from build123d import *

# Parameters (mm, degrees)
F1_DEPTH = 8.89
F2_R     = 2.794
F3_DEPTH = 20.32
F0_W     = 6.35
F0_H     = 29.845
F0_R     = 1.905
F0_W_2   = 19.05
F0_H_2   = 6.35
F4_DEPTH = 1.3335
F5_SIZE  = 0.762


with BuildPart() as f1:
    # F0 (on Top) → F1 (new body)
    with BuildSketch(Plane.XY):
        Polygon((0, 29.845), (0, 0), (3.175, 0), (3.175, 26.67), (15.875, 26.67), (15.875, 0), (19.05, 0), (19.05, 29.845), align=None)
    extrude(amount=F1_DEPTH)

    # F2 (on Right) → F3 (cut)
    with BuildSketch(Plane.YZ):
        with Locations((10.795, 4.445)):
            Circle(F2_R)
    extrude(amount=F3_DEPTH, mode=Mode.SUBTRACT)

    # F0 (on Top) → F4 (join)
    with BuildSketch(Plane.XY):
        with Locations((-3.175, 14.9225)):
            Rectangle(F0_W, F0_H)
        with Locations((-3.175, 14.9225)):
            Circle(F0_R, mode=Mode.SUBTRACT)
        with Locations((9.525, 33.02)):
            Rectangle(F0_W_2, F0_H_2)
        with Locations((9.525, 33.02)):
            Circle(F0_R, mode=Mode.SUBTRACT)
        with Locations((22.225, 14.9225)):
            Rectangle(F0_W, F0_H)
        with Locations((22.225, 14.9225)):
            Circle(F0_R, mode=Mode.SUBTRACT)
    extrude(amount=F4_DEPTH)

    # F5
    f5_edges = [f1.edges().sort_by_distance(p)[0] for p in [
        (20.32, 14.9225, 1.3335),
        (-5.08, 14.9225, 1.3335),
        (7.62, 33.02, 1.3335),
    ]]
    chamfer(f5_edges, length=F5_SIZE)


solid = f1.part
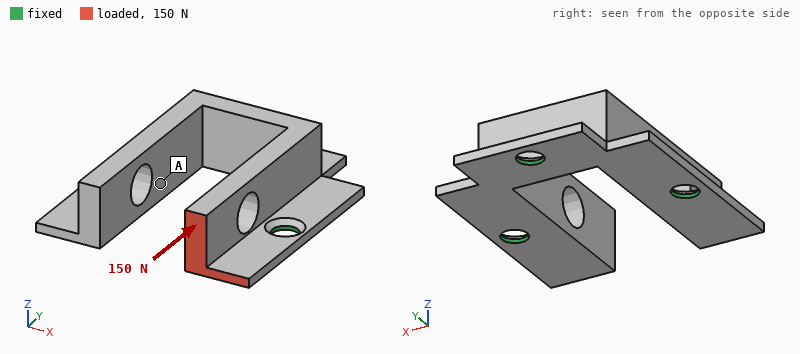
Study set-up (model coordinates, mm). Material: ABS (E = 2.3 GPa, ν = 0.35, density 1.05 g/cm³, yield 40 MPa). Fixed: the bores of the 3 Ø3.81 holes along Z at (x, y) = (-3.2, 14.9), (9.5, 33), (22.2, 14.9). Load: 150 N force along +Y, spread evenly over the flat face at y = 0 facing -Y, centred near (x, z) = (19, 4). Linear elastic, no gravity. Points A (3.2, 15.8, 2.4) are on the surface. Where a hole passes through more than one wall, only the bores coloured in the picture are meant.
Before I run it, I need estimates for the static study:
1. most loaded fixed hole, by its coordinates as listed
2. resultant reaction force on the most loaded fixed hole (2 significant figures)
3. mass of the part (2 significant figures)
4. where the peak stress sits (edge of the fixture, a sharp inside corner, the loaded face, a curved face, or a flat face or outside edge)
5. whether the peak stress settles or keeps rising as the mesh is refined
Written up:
(22.2, 14.9)
120 N
2.6 g
edge of the fixture
keeps rising
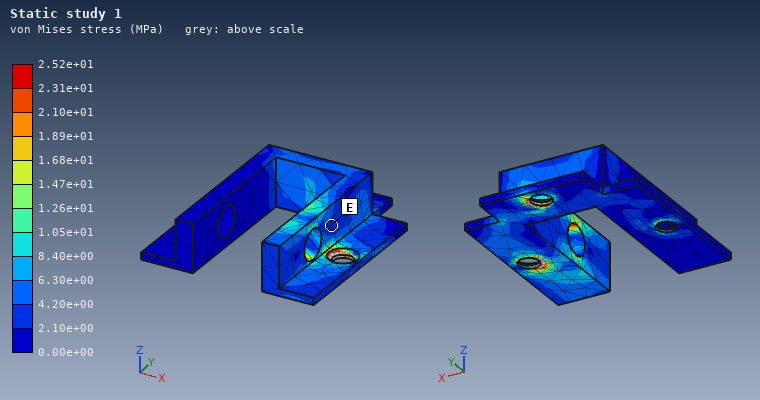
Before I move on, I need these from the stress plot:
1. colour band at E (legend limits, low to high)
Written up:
2.10e+00 to 4.20e+00 MPa
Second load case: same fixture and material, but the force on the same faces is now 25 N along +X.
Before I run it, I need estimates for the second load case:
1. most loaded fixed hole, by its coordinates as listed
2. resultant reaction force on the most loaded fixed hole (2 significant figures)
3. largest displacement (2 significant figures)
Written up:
(22.2, 14.9)
34 N
0.49 mm
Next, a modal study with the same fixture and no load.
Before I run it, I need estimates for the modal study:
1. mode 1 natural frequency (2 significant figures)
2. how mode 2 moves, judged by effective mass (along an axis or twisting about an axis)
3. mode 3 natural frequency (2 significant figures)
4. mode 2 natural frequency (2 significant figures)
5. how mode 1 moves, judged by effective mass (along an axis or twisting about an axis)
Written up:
1800 Hz
along Z
3300 Hz
2200 Hz
along X
